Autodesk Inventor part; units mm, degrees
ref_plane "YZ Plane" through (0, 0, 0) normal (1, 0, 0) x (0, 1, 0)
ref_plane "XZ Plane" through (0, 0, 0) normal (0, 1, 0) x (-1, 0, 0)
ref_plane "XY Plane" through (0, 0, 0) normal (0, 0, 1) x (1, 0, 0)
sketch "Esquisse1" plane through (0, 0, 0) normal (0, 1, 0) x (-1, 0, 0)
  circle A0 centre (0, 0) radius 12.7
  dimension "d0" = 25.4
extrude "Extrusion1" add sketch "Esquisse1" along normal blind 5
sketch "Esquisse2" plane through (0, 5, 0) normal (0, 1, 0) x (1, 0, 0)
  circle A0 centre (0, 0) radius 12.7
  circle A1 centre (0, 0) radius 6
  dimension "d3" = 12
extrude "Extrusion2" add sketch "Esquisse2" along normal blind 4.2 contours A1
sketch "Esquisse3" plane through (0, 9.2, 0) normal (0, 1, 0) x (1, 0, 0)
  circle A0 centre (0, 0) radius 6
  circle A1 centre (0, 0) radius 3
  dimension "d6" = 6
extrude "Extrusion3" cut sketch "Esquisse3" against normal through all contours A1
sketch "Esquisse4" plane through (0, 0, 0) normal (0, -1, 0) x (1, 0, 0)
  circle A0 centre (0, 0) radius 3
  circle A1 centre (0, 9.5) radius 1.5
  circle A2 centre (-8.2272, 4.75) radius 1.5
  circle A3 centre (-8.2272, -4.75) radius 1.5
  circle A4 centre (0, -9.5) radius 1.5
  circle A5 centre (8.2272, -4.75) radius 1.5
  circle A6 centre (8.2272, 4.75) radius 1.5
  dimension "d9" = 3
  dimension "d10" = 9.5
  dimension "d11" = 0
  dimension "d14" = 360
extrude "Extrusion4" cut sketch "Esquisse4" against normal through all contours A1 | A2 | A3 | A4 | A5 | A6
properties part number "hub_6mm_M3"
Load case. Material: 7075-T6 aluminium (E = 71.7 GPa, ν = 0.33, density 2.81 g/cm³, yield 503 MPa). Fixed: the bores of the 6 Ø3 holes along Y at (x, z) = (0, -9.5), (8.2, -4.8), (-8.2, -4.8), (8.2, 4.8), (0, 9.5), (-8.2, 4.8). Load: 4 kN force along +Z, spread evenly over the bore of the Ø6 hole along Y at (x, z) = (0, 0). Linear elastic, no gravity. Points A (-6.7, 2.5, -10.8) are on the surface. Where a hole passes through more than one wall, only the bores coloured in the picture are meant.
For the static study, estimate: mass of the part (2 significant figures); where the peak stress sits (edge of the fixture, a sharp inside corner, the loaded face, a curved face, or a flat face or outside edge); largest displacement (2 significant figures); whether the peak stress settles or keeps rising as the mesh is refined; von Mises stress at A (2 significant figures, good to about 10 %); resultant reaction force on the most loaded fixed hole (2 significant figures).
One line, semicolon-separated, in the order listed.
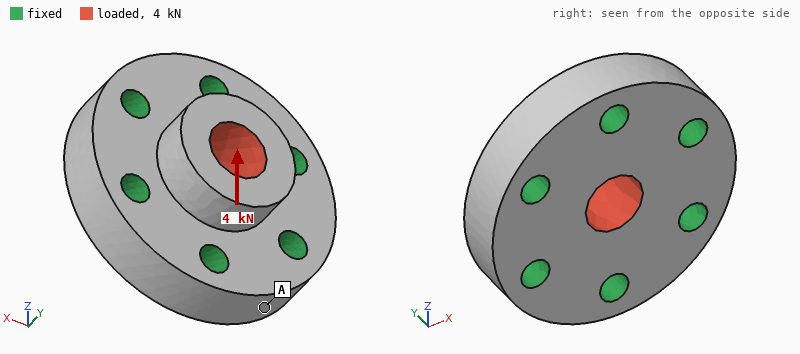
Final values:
7.1 g; a sharp inside corner; 8.1 µm; keeps rising; 8.8 MPa; 1.1 kN
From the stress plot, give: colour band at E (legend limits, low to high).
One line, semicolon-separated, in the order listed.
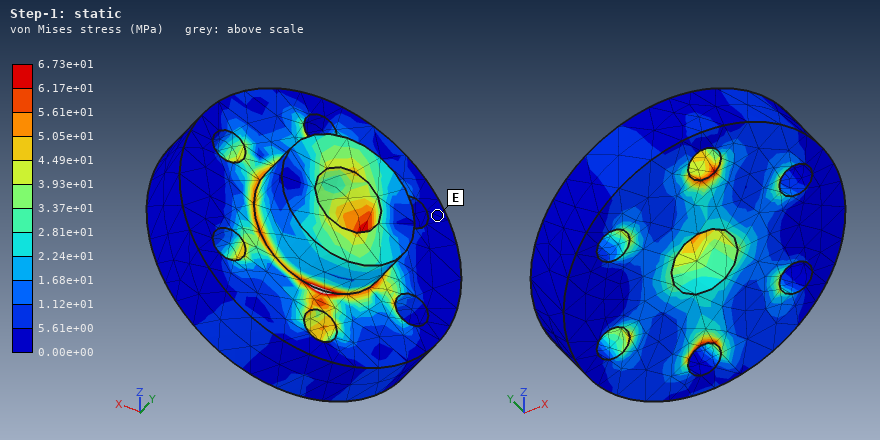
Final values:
0.00e+00 to 5.61e+00 MPa
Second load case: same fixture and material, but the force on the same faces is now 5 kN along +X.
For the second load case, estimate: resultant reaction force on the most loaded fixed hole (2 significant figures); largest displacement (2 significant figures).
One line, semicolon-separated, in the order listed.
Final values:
1.2 kN; 10 µm
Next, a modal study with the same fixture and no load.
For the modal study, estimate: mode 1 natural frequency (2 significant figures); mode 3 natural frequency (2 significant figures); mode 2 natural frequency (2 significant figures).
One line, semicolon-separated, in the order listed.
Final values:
92 kHz; 96 kHz; 95 kHz
